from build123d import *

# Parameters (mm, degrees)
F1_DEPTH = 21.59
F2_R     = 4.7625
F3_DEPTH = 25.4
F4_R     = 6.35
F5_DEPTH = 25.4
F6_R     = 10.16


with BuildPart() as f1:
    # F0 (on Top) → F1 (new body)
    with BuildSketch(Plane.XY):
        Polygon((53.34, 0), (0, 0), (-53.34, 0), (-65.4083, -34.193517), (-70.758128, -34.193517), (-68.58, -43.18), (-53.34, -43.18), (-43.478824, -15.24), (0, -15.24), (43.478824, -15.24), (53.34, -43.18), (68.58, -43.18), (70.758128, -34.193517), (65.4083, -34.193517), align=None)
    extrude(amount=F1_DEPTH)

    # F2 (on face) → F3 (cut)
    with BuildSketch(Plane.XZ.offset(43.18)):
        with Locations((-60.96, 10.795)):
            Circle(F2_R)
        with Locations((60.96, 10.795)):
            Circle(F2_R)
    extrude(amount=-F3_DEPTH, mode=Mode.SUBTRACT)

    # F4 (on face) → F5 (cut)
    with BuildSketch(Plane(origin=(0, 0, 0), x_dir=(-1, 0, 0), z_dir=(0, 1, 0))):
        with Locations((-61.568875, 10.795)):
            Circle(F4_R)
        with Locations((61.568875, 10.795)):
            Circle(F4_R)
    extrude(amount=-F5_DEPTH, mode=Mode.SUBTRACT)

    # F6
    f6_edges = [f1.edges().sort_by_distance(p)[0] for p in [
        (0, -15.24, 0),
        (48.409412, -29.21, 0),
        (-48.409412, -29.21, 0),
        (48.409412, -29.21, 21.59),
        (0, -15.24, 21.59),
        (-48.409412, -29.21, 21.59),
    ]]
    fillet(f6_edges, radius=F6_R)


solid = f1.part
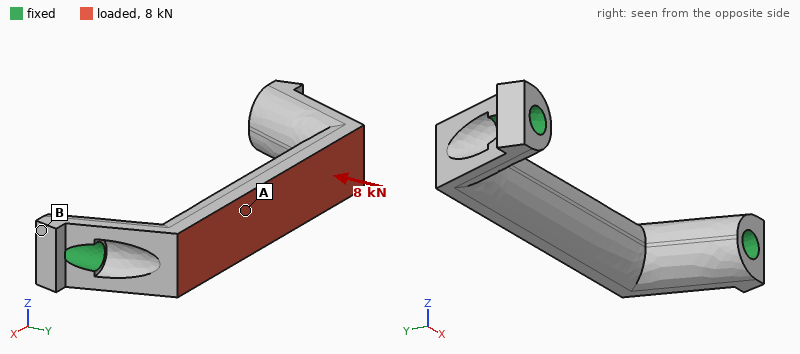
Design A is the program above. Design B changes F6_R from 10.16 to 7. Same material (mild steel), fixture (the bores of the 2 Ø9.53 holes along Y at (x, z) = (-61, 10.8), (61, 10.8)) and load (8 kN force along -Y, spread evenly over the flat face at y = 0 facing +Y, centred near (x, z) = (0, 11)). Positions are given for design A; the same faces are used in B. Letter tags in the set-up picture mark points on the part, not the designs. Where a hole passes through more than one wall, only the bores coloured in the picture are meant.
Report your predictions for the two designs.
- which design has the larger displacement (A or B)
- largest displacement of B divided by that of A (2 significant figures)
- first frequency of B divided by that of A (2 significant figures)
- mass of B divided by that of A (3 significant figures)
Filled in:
A
0.86
1.0
1.08
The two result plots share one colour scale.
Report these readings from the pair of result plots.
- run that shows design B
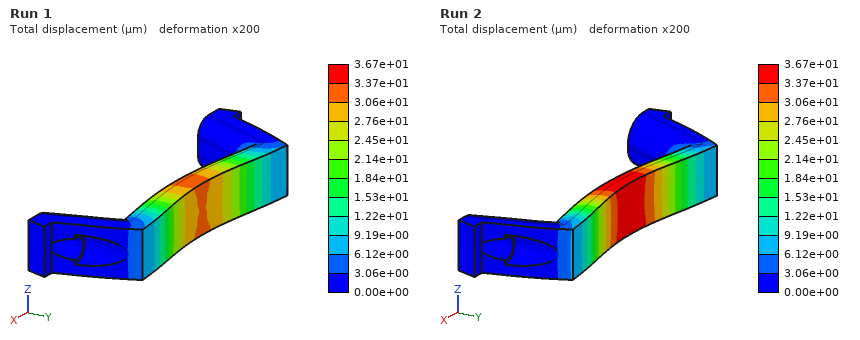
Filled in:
Run 1
